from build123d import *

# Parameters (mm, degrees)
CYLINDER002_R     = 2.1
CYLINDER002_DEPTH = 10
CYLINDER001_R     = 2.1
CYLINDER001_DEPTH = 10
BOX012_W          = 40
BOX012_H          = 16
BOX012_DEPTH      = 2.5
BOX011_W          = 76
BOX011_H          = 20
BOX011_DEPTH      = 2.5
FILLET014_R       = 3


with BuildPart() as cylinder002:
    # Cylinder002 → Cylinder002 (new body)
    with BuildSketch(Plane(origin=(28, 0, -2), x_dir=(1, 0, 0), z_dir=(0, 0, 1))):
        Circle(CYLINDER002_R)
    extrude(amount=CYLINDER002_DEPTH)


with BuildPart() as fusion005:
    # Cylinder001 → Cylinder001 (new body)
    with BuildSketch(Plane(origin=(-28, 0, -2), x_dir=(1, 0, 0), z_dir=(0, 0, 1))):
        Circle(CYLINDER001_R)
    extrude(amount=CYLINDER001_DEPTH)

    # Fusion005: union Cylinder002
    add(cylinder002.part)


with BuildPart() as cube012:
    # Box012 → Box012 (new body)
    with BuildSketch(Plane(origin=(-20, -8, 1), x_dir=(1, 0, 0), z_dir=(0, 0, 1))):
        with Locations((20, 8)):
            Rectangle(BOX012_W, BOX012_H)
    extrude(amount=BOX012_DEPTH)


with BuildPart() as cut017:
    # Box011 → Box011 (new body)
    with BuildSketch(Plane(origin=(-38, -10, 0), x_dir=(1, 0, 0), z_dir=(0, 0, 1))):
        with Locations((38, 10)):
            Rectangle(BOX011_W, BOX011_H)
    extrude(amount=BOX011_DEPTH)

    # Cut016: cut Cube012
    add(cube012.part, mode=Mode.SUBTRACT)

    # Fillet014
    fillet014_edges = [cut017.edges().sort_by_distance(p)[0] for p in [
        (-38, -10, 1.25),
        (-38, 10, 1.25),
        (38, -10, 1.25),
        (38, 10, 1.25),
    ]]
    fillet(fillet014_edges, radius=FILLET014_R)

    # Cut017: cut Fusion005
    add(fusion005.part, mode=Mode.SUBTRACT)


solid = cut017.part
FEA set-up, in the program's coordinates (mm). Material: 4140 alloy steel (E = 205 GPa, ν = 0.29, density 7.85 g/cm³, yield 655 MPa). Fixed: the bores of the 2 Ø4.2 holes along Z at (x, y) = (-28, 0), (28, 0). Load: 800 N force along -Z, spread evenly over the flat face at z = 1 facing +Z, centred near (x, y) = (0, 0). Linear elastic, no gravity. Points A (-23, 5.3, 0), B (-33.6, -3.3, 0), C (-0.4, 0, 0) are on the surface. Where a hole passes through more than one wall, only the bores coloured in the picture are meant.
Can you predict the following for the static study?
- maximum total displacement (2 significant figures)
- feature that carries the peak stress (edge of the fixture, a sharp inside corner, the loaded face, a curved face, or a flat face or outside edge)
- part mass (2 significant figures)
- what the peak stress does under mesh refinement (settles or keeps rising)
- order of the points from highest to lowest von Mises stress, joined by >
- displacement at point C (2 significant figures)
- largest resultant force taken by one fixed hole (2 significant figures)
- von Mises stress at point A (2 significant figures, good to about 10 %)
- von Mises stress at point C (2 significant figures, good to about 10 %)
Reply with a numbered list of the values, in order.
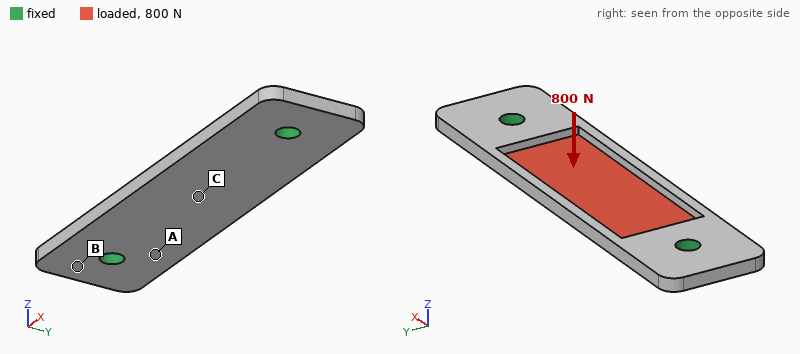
1. 0.19 mm
2. edge of the fixture
3. 22 g
4. keeps rising
5. C > A > B
6. 0.19 mm
7. 530 N
8. 130 MPa
9. 200 MPa
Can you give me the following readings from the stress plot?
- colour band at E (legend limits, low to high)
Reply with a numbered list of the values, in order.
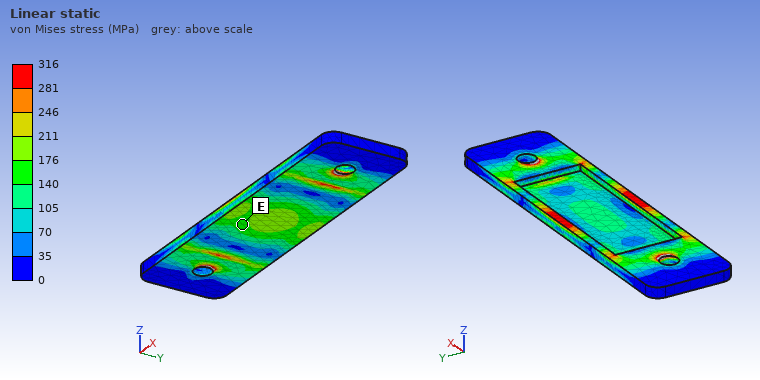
1. 140 to 176 MPa
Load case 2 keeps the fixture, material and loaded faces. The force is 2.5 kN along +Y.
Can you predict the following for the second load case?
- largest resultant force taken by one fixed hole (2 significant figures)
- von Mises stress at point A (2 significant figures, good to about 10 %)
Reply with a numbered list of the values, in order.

1. 1.3 kN
2. 40 MPa
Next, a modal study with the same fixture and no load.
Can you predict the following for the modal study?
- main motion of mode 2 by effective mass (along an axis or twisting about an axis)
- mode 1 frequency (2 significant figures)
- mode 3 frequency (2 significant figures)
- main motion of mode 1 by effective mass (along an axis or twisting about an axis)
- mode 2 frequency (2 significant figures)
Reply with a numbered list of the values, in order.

1. twisting about X
2. 4300 Hz
3. 10 kHz
4. along Z
5. 5700 Hz
